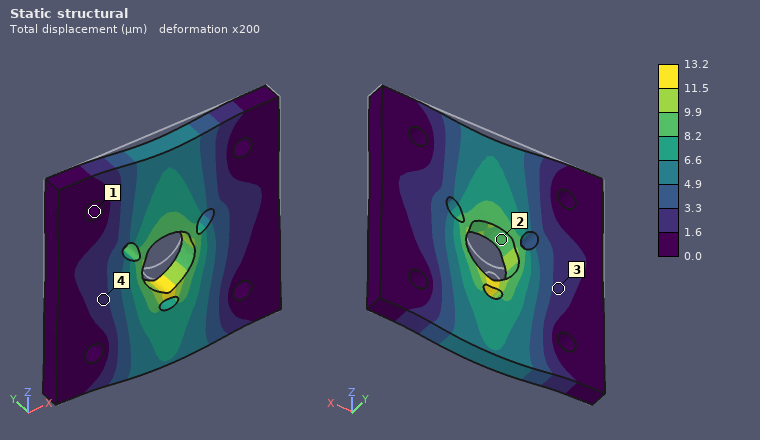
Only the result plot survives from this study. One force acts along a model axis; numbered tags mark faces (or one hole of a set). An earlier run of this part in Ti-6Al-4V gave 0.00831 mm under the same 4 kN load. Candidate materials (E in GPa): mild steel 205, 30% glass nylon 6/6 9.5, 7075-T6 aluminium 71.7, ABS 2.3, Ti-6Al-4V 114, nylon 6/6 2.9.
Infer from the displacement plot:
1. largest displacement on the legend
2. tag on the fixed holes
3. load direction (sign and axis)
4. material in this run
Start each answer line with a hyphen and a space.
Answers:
- 13.2 µm
- 1
- -Z
- 7075-T6 aluminium
